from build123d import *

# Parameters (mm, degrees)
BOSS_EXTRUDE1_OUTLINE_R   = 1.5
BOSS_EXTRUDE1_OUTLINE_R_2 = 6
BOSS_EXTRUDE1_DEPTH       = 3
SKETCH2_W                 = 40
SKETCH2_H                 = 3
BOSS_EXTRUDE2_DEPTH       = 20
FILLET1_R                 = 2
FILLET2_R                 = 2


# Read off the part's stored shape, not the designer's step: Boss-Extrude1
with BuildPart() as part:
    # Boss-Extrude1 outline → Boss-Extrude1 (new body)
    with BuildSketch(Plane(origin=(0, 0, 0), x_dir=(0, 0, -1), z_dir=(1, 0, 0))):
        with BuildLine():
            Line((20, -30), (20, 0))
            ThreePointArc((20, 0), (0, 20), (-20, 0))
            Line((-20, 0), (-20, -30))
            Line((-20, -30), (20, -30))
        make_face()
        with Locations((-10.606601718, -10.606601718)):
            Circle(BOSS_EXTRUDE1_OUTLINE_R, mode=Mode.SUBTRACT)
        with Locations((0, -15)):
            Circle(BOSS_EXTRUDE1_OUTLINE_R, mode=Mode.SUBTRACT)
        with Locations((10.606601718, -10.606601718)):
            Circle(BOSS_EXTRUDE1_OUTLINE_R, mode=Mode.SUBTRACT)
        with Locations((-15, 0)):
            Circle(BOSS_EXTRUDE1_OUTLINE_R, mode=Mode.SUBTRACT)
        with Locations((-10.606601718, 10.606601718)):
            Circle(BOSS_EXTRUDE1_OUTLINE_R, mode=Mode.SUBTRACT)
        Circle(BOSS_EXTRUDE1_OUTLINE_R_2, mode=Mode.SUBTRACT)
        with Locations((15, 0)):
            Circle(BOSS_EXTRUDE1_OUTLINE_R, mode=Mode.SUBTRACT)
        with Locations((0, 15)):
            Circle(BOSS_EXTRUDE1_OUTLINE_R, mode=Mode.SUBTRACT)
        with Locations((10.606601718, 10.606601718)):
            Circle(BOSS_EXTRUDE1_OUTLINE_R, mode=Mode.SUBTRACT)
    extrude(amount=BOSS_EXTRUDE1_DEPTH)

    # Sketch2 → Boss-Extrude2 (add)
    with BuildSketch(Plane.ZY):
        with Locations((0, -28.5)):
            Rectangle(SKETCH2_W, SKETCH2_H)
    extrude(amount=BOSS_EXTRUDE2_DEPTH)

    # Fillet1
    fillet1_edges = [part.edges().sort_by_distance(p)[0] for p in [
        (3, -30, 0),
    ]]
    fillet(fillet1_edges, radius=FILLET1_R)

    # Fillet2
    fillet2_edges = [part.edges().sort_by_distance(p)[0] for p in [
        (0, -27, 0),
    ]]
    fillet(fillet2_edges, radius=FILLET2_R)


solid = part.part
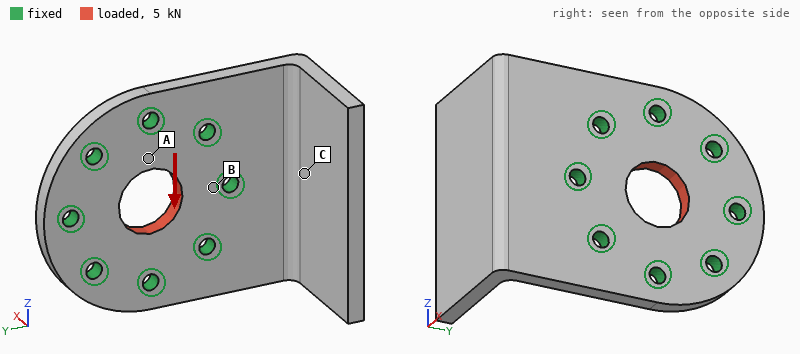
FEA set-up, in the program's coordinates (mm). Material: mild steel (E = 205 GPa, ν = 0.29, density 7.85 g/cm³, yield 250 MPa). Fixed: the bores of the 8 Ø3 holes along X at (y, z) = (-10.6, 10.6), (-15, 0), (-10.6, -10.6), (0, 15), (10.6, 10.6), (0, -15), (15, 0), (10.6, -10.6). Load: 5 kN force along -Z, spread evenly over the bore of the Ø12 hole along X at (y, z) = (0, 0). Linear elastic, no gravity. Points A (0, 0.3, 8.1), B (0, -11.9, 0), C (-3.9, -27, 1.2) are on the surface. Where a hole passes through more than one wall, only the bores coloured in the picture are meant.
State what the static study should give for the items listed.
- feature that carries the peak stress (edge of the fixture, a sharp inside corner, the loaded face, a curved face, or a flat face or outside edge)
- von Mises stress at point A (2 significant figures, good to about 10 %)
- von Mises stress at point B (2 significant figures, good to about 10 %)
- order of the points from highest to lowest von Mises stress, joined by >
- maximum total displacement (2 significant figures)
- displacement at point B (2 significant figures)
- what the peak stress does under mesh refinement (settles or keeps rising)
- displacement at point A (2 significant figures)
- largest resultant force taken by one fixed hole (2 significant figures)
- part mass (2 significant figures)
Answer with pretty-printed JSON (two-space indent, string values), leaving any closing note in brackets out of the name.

{
  "feature that carries the peak stress": "edge of the fixture",
  "von Mises stress at point A": "44 MPa",
  "von Mises stress at point B": "15 MPa",
  "order of the points from highest to lowest von Mises stress, joined by >": "A > B > C",
  "maximum total displacement": "2.0 µm",
  "displacement at point B": "0.30 µm",
  "what the peak stress does under mesh refinement": "keeps rising",
  "displacement at point A": "1.4 µm",
  "largest resultant force taken by one fixed hole": "1000 N",
  "part mass": "58 g"
}
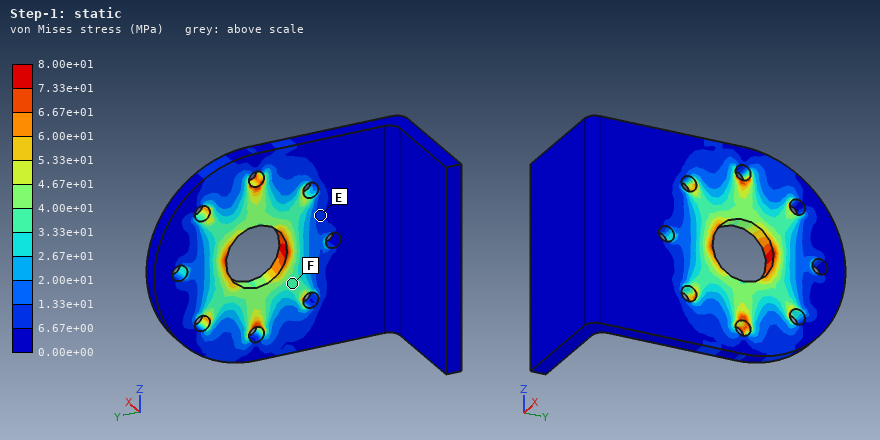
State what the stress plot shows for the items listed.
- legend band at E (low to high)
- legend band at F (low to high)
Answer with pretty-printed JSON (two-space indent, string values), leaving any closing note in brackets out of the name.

{
  "legend band at E": "6.67e+00 to 1.33e+01 MPa",
  "legend band at F": "3.33e+01 to 4.00e+01 MPa"
}
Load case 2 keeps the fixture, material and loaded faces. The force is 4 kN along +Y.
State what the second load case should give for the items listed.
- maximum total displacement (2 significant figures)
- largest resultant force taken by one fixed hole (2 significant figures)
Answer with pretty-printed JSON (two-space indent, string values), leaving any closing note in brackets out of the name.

{
  "maximum total displacement": "1.6 µm",
  "largest resultant force taken by one fixed hole": "800 N"
}
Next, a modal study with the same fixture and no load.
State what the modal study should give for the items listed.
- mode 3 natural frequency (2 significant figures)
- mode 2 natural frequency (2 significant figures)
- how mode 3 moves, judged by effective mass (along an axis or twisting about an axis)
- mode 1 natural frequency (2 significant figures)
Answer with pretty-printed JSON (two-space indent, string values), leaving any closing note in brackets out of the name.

{
  "mode 3 natural frequency": "7300 Hz",
  "mode 2 natural frequency": "3800 Hz",
  "how mode 3 moves, judged by effective mass": "along X",
  "mode 1 natural frequency": "2500 Hz"
}
